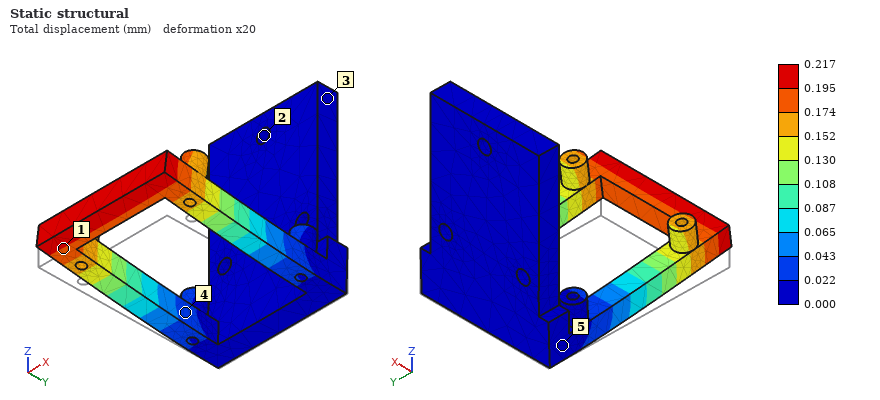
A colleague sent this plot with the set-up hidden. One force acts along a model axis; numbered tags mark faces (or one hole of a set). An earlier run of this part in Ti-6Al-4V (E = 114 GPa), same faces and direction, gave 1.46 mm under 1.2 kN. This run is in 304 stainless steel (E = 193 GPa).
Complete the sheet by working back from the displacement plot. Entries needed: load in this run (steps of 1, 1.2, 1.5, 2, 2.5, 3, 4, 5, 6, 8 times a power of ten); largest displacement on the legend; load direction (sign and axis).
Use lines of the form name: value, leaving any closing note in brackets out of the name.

load in this run: 300 N
largest displacement on the legend: 0.217 mm
load direction: +Z
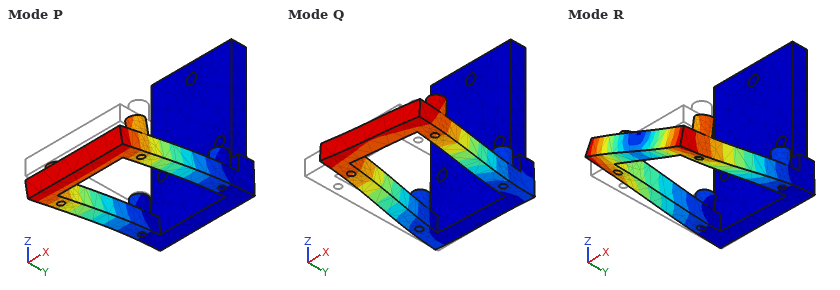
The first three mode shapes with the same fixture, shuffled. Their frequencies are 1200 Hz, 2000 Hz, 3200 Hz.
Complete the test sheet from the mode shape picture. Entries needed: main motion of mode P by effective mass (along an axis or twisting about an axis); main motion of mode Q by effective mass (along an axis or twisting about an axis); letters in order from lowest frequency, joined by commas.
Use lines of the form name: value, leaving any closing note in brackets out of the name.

main motion of mode P by effective mass: along Z
main motion of mode Q by effective mass: along X
letters in order from lowest frequency, joined by commas: P, Q, R
